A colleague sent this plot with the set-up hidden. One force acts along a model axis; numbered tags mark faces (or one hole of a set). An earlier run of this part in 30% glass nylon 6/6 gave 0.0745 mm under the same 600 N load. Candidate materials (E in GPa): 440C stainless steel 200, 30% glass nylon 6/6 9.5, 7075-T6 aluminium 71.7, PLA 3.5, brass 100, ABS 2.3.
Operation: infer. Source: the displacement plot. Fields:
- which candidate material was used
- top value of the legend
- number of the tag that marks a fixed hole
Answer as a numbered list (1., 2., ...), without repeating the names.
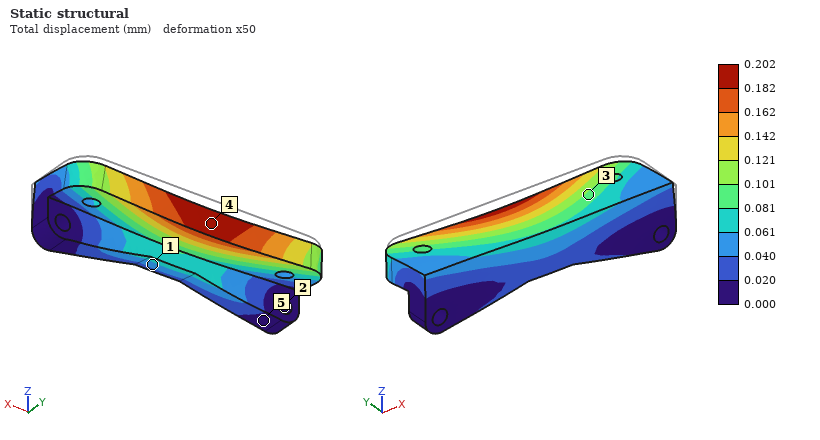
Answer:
1. PLA
2. 0.202 mm
3. 2
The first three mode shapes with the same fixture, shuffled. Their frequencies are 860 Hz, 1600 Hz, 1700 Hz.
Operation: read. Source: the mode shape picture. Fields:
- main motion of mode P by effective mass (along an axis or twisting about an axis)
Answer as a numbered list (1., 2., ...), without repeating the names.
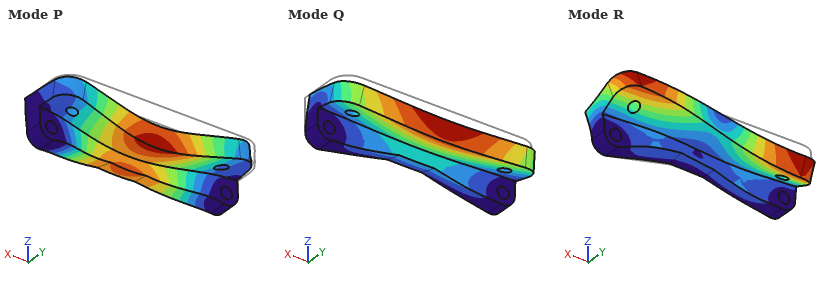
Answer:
1. along Y
